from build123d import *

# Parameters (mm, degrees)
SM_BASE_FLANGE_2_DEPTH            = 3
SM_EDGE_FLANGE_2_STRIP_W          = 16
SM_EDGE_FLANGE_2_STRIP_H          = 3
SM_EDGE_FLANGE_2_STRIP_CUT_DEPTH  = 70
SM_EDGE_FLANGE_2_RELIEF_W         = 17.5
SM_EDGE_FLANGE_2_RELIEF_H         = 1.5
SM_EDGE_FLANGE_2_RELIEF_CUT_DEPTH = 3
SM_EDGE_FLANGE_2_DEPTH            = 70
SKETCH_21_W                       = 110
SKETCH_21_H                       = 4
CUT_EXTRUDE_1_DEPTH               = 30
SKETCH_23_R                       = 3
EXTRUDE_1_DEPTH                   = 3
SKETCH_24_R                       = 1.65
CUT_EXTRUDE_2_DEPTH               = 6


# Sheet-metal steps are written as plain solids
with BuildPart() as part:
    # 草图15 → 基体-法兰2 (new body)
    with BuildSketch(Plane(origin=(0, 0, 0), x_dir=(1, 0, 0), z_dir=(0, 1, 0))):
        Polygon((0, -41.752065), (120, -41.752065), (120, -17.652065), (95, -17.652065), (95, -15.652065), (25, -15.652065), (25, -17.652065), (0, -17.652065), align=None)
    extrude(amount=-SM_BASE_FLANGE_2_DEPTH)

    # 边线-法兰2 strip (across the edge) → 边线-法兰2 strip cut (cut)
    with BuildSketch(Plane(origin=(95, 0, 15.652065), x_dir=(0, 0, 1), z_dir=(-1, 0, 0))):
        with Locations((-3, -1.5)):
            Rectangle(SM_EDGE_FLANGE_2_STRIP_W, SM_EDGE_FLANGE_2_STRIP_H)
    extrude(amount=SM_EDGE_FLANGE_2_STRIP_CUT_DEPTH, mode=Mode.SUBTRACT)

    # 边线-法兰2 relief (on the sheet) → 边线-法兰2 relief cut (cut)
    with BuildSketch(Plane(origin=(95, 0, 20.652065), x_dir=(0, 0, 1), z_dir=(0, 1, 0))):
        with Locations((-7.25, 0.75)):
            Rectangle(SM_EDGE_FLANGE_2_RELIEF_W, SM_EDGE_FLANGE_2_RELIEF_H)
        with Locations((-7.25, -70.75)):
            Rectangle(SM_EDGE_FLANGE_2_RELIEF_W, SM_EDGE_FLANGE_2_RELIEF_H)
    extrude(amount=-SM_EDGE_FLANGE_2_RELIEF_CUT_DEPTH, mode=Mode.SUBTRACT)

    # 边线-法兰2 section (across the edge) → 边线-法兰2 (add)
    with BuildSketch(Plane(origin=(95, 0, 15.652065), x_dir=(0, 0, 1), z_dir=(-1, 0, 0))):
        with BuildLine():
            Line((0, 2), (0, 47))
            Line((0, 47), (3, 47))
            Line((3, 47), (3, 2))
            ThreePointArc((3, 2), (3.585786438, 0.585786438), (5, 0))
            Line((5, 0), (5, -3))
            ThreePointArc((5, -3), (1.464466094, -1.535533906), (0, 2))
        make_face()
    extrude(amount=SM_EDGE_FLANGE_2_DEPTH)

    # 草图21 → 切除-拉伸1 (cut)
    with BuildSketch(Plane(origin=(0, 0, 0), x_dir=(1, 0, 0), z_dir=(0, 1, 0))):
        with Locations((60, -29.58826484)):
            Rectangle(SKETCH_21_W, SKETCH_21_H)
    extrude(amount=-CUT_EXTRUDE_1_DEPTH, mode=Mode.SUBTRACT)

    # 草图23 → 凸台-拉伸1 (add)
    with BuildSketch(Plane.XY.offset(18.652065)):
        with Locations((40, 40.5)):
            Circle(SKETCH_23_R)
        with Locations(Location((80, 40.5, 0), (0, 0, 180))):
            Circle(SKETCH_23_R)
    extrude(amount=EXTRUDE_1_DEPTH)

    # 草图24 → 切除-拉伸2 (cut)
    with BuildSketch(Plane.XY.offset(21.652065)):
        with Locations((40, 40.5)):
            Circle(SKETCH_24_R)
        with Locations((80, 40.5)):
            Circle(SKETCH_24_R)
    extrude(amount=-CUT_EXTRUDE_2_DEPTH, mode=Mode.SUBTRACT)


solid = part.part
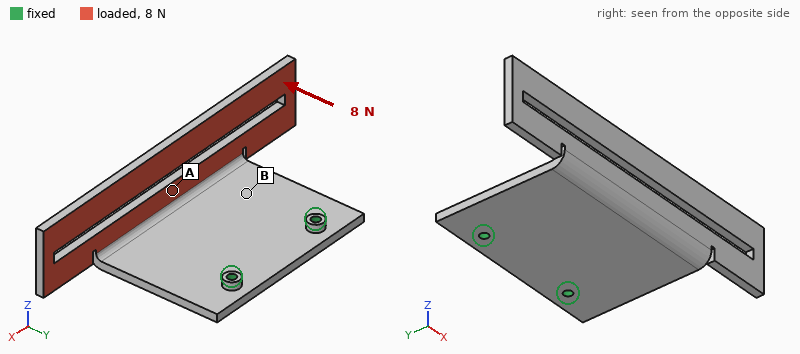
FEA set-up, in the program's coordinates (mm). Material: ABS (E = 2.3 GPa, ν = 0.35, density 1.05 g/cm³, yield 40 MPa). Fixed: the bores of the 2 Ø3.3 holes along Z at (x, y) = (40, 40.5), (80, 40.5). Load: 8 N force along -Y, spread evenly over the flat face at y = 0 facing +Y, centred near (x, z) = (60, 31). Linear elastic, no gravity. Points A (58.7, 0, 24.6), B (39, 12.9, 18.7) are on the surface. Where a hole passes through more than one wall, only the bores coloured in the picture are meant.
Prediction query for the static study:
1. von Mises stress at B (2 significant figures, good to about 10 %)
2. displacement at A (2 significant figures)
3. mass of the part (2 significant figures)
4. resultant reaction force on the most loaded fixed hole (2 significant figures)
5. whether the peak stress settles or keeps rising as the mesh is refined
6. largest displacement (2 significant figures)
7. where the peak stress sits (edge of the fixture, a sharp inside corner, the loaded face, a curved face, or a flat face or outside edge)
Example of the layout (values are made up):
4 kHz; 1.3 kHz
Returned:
1.0 MPa; 0.27 mm; 18 g; 4.1 N; keeps rising; 1.5 mm; a sharp inside corner
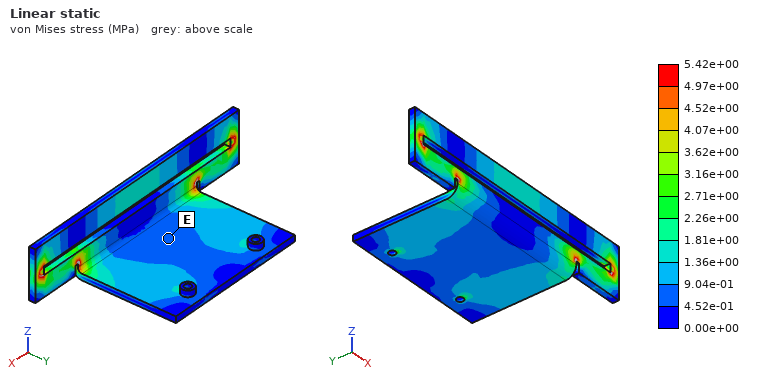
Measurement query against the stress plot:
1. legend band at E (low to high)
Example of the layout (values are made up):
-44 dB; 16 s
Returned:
4.52e-01 to 9.04e-01 MPa
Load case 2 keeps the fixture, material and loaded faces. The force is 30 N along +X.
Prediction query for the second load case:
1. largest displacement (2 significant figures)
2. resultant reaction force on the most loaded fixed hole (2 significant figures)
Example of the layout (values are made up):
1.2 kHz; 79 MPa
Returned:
1.4 mm; 34 N
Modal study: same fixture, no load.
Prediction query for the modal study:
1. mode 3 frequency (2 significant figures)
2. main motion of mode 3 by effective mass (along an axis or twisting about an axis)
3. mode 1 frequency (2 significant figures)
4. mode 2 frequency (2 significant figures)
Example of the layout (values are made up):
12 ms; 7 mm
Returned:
220 Hz; along Z; 150 Hz; 210 Hz
